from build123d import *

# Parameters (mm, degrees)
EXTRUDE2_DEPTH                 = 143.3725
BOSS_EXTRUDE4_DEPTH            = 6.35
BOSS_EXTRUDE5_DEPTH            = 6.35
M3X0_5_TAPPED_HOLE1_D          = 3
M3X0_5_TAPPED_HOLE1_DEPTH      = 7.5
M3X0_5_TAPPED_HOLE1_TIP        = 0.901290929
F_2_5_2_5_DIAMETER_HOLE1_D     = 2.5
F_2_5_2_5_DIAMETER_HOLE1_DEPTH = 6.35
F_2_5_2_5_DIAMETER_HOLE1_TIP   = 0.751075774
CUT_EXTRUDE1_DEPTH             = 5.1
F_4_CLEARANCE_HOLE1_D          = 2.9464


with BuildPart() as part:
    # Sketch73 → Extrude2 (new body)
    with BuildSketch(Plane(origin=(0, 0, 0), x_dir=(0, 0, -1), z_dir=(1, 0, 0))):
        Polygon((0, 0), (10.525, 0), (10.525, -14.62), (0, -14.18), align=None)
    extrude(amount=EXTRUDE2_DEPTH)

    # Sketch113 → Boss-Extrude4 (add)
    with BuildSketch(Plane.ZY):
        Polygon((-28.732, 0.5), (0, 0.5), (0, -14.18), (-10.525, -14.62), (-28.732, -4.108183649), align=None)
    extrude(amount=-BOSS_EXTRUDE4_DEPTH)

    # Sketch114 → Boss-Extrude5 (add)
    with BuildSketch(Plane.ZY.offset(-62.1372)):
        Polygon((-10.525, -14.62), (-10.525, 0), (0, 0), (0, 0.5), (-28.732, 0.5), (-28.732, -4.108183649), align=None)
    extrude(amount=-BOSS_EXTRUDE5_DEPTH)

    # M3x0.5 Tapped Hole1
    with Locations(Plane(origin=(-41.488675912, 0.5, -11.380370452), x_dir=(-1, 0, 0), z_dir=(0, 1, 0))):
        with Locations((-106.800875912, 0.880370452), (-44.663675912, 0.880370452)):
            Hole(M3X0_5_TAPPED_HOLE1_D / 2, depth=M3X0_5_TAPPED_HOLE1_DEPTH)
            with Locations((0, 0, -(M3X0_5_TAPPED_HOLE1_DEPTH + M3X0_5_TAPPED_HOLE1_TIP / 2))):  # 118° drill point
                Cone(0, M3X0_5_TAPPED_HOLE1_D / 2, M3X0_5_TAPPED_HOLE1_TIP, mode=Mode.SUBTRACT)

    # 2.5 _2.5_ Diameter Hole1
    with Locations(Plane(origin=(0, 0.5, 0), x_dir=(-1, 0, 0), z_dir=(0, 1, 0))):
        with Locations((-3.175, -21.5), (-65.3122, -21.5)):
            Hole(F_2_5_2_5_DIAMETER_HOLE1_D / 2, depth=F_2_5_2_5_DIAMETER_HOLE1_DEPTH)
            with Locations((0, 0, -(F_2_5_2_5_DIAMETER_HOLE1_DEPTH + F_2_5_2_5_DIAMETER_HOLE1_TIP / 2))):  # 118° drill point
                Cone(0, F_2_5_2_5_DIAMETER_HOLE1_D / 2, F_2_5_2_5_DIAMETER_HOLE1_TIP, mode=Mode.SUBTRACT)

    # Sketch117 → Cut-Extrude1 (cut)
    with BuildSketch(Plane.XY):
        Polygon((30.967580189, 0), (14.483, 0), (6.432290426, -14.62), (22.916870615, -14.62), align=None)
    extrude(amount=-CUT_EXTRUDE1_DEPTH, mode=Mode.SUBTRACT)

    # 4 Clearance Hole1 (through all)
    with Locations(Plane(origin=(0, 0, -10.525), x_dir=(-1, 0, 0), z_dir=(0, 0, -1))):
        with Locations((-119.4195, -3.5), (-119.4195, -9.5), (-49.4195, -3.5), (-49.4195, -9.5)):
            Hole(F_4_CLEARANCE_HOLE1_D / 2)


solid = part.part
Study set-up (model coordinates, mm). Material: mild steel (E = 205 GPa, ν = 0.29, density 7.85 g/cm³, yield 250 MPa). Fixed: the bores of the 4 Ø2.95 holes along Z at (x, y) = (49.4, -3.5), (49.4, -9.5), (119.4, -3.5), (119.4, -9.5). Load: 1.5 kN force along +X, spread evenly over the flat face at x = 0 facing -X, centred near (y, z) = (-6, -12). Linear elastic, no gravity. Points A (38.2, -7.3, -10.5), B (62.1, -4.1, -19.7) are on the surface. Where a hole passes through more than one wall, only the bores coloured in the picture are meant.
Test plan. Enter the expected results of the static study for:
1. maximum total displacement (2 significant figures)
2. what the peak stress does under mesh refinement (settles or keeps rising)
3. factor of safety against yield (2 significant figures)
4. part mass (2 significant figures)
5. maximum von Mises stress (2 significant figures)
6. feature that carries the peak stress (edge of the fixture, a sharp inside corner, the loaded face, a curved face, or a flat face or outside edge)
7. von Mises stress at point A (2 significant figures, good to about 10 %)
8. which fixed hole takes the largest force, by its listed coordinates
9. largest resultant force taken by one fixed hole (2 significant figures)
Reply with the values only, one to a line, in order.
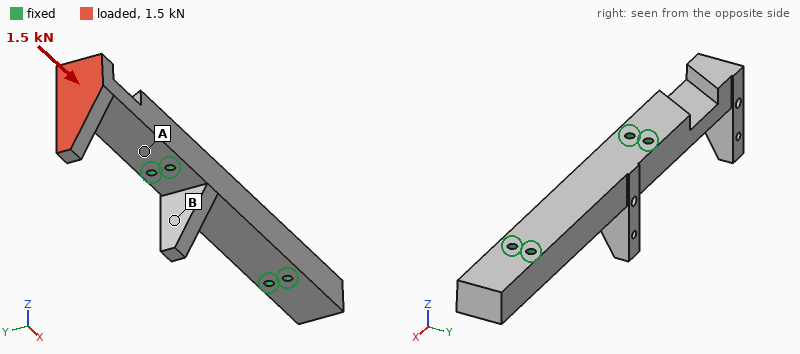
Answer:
0.14 mm
settles
2.0
180 g
130 MPa
a flat face or outside edge
49 MPa
(49.4, -3.5)
890 N
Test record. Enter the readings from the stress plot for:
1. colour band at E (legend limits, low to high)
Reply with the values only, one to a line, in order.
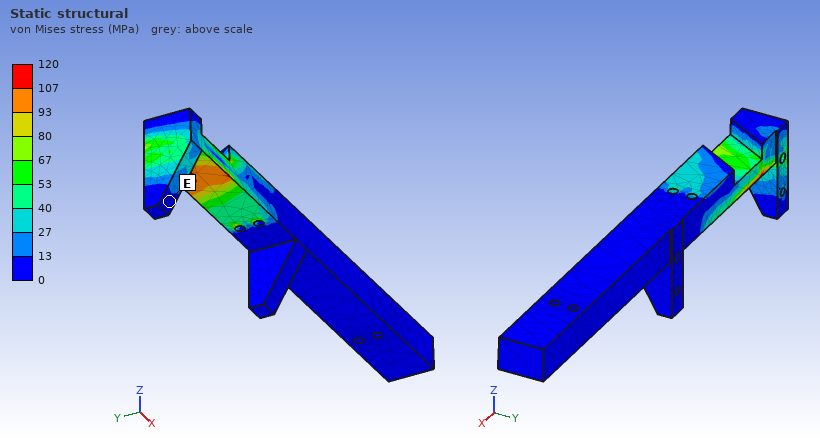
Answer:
0 to 13 MPa
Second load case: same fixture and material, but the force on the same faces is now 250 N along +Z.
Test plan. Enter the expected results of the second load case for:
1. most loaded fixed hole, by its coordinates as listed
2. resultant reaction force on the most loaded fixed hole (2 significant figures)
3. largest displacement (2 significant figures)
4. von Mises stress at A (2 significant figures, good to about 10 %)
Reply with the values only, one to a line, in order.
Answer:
(49.4, -3.5)
140 N
0.10 mm
37 MPa
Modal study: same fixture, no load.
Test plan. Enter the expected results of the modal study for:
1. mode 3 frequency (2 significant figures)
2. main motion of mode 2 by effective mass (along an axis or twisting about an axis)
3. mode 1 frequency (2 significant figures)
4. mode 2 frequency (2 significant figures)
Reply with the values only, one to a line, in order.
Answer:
6200 Hz
along Y
2100 Hz
3500 Hz
